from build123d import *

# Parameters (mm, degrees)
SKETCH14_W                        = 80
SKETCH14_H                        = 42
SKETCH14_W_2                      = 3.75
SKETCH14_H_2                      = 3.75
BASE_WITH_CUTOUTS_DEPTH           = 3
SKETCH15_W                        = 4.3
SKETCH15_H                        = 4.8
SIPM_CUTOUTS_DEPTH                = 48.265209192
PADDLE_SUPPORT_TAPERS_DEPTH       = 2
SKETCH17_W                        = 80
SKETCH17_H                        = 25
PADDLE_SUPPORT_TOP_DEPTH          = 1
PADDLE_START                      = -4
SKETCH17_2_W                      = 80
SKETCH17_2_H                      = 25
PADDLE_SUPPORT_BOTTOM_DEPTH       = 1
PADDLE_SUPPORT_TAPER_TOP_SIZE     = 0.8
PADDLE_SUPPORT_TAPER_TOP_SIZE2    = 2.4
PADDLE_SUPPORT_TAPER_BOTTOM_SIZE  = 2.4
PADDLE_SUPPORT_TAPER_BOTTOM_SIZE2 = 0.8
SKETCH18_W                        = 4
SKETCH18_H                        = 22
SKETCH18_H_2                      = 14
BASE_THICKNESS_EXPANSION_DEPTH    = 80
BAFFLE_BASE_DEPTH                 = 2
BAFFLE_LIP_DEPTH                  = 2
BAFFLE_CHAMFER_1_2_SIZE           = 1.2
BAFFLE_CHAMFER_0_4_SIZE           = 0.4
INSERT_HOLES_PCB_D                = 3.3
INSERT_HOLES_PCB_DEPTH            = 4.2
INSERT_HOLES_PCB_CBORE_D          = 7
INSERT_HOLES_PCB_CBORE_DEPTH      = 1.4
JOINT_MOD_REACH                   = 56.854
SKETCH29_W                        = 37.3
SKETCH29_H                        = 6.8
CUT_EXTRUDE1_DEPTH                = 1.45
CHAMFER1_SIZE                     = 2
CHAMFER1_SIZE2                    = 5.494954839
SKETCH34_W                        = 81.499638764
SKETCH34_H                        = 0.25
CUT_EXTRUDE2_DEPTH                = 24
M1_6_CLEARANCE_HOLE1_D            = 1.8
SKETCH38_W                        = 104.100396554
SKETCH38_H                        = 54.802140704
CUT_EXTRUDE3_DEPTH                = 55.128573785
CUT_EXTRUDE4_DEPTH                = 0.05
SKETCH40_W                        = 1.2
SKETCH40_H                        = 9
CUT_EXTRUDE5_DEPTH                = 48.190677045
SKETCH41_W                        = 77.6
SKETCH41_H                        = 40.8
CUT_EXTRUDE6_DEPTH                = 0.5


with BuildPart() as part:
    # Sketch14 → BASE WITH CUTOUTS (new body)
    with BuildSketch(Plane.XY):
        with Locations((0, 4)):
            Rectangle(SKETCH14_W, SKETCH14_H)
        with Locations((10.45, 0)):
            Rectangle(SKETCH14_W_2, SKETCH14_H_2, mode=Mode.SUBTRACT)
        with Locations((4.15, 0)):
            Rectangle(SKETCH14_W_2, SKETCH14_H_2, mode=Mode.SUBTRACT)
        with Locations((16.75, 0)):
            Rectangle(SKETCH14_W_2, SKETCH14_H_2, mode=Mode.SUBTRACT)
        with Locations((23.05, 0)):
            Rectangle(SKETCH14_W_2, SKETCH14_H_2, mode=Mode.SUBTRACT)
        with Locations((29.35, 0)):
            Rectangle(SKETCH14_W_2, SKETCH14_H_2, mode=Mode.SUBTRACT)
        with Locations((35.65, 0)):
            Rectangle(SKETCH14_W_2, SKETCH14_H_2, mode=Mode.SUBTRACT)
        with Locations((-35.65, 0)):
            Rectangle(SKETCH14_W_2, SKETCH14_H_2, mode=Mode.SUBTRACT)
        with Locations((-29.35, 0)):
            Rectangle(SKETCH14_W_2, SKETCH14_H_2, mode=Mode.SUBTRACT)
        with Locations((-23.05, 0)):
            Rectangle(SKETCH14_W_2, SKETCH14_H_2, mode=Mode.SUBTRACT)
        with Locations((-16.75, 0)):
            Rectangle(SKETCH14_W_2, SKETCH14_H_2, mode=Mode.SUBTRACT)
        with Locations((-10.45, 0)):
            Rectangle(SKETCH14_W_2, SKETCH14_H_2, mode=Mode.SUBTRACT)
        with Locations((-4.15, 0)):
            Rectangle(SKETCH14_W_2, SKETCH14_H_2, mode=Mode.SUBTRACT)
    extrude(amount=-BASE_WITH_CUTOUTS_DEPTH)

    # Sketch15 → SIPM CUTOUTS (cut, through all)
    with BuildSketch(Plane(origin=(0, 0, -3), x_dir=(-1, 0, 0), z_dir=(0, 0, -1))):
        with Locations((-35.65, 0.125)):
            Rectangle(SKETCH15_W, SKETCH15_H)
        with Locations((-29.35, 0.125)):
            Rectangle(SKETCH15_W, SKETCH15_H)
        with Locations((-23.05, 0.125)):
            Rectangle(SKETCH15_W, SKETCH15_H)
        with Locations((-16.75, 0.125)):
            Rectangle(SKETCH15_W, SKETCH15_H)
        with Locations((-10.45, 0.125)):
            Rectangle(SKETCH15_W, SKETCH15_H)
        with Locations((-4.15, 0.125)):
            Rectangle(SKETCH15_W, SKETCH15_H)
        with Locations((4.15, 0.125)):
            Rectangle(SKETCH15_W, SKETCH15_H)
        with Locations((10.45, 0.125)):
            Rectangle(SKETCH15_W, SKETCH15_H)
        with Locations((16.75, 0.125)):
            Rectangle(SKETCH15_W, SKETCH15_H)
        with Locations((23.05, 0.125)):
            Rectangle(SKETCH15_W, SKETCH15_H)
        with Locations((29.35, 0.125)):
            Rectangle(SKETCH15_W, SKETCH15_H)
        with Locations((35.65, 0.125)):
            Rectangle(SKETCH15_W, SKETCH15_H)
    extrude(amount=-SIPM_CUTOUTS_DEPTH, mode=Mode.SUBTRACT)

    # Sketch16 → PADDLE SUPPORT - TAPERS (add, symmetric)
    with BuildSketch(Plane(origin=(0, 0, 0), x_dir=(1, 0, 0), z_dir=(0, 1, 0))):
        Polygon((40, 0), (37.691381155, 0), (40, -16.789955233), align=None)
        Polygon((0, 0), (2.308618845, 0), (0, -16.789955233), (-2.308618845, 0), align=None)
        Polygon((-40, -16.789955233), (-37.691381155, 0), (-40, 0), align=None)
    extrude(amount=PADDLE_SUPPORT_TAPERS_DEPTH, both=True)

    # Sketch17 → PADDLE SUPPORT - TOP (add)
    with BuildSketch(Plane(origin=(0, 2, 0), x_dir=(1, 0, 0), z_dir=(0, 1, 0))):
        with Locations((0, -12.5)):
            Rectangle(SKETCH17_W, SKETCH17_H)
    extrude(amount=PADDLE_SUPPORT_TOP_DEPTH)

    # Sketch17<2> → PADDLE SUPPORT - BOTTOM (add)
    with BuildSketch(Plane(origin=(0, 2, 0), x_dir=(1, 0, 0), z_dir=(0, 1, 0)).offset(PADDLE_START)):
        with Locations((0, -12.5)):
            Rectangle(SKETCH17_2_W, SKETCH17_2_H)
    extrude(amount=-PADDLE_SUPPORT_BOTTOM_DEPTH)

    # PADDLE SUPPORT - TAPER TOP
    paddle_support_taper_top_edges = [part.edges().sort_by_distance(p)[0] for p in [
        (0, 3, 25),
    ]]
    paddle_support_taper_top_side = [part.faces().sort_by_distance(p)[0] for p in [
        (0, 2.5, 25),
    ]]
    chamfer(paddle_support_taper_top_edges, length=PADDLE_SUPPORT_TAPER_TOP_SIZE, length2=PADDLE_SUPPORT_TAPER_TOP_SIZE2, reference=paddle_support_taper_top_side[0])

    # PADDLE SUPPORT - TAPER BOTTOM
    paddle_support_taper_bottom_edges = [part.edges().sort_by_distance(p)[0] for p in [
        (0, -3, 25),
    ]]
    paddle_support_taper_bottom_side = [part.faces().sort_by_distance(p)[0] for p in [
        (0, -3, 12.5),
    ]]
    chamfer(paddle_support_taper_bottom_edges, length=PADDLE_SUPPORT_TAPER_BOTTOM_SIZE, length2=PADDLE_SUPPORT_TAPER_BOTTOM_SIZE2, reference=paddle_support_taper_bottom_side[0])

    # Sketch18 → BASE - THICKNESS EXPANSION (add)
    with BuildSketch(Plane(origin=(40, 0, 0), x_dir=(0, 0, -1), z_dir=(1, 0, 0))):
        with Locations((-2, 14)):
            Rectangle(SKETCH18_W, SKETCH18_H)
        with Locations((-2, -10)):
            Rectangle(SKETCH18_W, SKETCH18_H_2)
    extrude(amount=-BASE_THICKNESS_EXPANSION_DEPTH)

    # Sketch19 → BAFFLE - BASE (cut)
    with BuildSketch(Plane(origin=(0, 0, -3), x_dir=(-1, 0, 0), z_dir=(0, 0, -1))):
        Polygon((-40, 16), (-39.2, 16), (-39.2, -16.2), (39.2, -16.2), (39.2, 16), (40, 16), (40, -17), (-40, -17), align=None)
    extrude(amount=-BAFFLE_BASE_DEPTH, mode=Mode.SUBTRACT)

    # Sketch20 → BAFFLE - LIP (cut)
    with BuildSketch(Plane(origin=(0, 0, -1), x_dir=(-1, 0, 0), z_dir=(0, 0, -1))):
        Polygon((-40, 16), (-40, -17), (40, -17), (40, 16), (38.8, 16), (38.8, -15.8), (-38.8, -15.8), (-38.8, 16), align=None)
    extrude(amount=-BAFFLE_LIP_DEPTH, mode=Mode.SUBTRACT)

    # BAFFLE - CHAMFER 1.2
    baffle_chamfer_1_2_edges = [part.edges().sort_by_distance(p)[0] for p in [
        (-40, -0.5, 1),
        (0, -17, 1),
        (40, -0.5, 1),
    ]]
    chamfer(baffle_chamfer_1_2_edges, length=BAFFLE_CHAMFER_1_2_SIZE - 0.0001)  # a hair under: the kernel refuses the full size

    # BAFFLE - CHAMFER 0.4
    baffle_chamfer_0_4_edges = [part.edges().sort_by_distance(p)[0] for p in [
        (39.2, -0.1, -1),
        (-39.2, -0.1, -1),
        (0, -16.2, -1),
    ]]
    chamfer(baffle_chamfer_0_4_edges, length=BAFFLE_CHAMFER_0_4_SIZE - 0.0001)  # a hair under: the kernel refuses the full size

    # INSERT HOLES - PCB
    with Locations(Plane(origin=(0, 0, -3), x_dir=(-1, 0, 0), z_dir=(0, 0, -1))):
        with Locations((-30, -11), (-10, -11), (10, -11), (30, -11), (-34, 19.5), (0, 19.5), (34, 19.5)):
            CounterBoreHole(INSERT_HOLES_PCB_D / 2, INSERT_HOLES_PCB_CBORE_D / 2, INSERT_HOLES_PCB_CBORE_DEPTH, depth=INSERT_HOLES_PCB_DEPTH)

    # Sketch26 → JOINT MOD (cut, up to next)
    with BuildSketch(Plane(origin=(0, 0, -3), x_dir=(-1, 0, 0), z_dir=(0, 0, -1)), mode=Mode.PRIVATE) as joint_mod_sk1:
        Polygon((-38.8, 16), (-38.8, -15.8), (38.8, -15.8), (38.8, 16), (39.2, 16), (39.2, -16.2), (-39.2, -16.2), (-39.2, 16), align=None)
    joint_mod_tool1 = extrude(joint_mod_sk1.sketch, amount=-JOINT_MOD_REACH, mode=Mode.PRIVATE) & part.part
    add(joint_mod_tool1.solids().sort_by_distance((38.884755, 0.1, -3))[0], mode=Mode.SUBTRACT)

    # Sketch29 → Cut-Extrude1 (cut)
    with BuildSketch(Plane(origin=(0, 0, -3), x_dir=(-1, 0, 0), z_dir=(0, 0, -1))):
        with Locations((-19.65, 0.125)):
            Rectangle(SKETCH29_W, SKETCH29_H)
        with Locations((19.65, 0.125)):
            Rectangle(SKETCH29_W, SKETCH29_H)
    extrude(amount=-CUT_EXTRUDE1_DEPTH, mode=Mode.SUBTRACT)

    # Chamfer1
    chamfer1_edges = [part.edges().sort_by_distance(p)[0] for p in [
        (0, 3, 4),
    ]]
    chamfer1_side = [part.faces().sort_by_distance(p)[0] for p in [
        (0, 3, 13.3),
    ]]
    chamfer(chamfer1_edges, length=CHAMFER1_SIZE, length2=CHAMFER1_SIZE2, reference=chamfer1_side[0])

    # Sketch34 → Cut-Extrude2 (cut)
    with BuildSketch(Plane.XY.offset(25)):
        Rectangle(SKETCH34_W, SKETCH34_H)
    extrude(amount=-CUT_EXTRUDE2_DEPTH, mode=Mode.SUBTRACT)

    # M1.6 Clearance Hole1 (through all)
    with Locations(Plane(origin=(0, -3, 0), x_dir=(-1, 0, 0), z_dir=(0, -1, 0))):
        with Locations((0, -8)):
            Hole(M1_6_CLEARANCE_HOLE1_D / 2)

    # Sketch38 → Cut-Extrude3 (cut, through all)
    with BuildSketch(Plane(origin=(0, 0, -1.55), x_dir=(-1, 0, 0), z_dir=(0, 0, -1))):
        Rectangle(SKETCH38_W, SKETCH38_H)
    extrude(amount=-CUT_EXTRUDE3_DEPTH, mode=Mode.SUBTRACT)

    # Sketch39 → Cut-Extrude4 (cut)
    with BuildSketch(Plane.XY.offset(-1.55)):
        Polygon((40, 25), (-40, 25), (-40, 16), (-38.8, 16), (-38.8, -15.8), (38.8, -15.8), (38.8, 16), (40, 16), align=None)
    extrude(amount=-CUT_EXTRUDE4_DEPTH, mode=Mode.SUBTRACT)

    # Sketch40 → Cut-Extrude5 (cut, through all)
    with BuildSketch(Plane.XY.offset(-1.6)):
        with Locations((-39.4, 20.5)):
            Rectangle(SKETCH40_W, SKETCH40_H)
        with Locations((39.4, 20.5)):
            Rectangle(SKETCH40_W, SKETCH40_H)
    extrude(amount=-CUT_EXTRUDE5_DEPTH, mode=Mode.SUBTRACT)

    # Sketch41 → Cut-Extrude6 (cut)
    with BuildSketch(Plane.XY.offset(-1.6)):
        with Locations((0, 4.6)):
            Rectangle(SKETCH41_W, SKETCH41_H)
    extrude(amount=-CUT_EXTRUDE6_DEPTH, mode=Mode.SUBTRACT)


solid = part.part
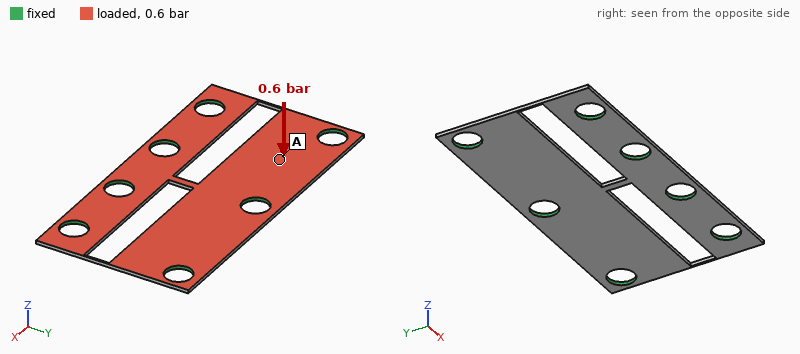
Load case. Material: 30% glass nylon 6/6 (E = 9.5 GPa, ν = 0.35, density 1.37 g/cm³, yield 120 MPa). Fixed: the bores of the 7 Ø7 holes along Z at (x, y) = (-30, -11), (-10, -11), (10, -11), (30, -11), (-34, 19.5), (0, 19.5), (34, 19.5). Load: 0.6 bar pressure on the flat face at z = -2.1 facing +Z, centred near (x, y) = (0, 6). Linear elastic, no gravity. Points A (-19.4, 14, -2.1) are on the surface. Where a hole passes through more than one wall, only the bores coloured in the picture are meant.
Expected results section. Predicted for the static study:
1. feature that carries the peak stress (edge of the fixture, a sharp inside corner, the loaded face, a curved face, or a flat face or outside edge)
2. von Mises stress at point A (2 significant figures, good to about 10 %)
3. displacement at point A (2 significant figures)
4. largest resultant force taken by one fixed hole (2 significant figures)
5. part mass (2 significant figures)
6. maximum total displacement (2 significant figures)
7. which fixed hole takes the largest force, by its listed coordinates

a flat face or outside edge
17 MPa
0.30 mm
39 N
2.9 g
0.67 mm
(0, 19.5)
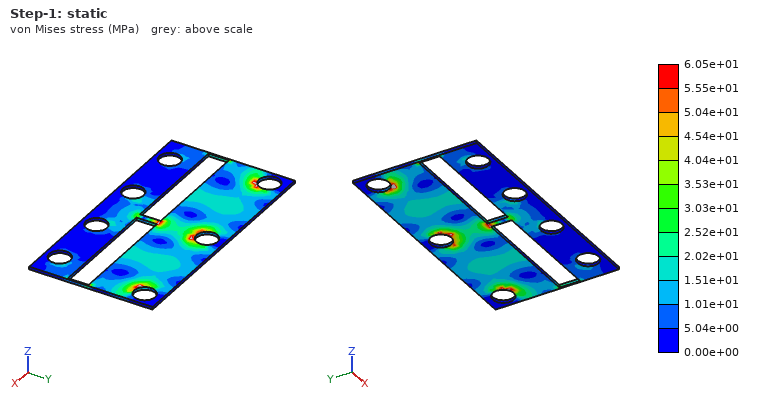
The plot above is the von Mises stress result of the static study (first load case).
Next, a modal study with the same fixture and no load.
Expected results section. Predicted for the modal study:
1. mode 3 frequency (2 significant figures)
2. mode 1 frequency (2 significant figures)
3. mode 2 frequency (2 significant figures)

3300 Hz
1800 Hz
1800 Hz
